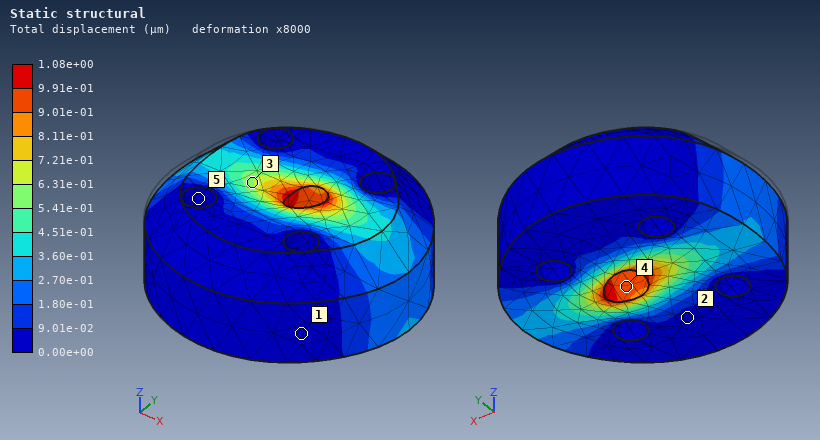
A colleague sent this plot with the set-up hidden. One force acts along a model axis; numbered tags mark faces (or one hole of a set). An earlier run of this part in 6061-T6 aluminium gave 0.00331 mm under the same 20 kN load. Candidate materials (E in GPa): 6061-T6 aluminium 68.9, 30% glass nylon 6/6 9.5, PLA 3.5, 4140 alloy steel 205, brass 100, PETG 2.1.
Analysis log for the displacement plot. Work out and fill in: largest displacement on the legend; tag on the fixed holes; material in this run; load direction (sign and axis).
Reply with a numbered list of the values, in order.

1. 1.08e+00 µm
2. 5
3. 4140 alloy steel
4. +X
